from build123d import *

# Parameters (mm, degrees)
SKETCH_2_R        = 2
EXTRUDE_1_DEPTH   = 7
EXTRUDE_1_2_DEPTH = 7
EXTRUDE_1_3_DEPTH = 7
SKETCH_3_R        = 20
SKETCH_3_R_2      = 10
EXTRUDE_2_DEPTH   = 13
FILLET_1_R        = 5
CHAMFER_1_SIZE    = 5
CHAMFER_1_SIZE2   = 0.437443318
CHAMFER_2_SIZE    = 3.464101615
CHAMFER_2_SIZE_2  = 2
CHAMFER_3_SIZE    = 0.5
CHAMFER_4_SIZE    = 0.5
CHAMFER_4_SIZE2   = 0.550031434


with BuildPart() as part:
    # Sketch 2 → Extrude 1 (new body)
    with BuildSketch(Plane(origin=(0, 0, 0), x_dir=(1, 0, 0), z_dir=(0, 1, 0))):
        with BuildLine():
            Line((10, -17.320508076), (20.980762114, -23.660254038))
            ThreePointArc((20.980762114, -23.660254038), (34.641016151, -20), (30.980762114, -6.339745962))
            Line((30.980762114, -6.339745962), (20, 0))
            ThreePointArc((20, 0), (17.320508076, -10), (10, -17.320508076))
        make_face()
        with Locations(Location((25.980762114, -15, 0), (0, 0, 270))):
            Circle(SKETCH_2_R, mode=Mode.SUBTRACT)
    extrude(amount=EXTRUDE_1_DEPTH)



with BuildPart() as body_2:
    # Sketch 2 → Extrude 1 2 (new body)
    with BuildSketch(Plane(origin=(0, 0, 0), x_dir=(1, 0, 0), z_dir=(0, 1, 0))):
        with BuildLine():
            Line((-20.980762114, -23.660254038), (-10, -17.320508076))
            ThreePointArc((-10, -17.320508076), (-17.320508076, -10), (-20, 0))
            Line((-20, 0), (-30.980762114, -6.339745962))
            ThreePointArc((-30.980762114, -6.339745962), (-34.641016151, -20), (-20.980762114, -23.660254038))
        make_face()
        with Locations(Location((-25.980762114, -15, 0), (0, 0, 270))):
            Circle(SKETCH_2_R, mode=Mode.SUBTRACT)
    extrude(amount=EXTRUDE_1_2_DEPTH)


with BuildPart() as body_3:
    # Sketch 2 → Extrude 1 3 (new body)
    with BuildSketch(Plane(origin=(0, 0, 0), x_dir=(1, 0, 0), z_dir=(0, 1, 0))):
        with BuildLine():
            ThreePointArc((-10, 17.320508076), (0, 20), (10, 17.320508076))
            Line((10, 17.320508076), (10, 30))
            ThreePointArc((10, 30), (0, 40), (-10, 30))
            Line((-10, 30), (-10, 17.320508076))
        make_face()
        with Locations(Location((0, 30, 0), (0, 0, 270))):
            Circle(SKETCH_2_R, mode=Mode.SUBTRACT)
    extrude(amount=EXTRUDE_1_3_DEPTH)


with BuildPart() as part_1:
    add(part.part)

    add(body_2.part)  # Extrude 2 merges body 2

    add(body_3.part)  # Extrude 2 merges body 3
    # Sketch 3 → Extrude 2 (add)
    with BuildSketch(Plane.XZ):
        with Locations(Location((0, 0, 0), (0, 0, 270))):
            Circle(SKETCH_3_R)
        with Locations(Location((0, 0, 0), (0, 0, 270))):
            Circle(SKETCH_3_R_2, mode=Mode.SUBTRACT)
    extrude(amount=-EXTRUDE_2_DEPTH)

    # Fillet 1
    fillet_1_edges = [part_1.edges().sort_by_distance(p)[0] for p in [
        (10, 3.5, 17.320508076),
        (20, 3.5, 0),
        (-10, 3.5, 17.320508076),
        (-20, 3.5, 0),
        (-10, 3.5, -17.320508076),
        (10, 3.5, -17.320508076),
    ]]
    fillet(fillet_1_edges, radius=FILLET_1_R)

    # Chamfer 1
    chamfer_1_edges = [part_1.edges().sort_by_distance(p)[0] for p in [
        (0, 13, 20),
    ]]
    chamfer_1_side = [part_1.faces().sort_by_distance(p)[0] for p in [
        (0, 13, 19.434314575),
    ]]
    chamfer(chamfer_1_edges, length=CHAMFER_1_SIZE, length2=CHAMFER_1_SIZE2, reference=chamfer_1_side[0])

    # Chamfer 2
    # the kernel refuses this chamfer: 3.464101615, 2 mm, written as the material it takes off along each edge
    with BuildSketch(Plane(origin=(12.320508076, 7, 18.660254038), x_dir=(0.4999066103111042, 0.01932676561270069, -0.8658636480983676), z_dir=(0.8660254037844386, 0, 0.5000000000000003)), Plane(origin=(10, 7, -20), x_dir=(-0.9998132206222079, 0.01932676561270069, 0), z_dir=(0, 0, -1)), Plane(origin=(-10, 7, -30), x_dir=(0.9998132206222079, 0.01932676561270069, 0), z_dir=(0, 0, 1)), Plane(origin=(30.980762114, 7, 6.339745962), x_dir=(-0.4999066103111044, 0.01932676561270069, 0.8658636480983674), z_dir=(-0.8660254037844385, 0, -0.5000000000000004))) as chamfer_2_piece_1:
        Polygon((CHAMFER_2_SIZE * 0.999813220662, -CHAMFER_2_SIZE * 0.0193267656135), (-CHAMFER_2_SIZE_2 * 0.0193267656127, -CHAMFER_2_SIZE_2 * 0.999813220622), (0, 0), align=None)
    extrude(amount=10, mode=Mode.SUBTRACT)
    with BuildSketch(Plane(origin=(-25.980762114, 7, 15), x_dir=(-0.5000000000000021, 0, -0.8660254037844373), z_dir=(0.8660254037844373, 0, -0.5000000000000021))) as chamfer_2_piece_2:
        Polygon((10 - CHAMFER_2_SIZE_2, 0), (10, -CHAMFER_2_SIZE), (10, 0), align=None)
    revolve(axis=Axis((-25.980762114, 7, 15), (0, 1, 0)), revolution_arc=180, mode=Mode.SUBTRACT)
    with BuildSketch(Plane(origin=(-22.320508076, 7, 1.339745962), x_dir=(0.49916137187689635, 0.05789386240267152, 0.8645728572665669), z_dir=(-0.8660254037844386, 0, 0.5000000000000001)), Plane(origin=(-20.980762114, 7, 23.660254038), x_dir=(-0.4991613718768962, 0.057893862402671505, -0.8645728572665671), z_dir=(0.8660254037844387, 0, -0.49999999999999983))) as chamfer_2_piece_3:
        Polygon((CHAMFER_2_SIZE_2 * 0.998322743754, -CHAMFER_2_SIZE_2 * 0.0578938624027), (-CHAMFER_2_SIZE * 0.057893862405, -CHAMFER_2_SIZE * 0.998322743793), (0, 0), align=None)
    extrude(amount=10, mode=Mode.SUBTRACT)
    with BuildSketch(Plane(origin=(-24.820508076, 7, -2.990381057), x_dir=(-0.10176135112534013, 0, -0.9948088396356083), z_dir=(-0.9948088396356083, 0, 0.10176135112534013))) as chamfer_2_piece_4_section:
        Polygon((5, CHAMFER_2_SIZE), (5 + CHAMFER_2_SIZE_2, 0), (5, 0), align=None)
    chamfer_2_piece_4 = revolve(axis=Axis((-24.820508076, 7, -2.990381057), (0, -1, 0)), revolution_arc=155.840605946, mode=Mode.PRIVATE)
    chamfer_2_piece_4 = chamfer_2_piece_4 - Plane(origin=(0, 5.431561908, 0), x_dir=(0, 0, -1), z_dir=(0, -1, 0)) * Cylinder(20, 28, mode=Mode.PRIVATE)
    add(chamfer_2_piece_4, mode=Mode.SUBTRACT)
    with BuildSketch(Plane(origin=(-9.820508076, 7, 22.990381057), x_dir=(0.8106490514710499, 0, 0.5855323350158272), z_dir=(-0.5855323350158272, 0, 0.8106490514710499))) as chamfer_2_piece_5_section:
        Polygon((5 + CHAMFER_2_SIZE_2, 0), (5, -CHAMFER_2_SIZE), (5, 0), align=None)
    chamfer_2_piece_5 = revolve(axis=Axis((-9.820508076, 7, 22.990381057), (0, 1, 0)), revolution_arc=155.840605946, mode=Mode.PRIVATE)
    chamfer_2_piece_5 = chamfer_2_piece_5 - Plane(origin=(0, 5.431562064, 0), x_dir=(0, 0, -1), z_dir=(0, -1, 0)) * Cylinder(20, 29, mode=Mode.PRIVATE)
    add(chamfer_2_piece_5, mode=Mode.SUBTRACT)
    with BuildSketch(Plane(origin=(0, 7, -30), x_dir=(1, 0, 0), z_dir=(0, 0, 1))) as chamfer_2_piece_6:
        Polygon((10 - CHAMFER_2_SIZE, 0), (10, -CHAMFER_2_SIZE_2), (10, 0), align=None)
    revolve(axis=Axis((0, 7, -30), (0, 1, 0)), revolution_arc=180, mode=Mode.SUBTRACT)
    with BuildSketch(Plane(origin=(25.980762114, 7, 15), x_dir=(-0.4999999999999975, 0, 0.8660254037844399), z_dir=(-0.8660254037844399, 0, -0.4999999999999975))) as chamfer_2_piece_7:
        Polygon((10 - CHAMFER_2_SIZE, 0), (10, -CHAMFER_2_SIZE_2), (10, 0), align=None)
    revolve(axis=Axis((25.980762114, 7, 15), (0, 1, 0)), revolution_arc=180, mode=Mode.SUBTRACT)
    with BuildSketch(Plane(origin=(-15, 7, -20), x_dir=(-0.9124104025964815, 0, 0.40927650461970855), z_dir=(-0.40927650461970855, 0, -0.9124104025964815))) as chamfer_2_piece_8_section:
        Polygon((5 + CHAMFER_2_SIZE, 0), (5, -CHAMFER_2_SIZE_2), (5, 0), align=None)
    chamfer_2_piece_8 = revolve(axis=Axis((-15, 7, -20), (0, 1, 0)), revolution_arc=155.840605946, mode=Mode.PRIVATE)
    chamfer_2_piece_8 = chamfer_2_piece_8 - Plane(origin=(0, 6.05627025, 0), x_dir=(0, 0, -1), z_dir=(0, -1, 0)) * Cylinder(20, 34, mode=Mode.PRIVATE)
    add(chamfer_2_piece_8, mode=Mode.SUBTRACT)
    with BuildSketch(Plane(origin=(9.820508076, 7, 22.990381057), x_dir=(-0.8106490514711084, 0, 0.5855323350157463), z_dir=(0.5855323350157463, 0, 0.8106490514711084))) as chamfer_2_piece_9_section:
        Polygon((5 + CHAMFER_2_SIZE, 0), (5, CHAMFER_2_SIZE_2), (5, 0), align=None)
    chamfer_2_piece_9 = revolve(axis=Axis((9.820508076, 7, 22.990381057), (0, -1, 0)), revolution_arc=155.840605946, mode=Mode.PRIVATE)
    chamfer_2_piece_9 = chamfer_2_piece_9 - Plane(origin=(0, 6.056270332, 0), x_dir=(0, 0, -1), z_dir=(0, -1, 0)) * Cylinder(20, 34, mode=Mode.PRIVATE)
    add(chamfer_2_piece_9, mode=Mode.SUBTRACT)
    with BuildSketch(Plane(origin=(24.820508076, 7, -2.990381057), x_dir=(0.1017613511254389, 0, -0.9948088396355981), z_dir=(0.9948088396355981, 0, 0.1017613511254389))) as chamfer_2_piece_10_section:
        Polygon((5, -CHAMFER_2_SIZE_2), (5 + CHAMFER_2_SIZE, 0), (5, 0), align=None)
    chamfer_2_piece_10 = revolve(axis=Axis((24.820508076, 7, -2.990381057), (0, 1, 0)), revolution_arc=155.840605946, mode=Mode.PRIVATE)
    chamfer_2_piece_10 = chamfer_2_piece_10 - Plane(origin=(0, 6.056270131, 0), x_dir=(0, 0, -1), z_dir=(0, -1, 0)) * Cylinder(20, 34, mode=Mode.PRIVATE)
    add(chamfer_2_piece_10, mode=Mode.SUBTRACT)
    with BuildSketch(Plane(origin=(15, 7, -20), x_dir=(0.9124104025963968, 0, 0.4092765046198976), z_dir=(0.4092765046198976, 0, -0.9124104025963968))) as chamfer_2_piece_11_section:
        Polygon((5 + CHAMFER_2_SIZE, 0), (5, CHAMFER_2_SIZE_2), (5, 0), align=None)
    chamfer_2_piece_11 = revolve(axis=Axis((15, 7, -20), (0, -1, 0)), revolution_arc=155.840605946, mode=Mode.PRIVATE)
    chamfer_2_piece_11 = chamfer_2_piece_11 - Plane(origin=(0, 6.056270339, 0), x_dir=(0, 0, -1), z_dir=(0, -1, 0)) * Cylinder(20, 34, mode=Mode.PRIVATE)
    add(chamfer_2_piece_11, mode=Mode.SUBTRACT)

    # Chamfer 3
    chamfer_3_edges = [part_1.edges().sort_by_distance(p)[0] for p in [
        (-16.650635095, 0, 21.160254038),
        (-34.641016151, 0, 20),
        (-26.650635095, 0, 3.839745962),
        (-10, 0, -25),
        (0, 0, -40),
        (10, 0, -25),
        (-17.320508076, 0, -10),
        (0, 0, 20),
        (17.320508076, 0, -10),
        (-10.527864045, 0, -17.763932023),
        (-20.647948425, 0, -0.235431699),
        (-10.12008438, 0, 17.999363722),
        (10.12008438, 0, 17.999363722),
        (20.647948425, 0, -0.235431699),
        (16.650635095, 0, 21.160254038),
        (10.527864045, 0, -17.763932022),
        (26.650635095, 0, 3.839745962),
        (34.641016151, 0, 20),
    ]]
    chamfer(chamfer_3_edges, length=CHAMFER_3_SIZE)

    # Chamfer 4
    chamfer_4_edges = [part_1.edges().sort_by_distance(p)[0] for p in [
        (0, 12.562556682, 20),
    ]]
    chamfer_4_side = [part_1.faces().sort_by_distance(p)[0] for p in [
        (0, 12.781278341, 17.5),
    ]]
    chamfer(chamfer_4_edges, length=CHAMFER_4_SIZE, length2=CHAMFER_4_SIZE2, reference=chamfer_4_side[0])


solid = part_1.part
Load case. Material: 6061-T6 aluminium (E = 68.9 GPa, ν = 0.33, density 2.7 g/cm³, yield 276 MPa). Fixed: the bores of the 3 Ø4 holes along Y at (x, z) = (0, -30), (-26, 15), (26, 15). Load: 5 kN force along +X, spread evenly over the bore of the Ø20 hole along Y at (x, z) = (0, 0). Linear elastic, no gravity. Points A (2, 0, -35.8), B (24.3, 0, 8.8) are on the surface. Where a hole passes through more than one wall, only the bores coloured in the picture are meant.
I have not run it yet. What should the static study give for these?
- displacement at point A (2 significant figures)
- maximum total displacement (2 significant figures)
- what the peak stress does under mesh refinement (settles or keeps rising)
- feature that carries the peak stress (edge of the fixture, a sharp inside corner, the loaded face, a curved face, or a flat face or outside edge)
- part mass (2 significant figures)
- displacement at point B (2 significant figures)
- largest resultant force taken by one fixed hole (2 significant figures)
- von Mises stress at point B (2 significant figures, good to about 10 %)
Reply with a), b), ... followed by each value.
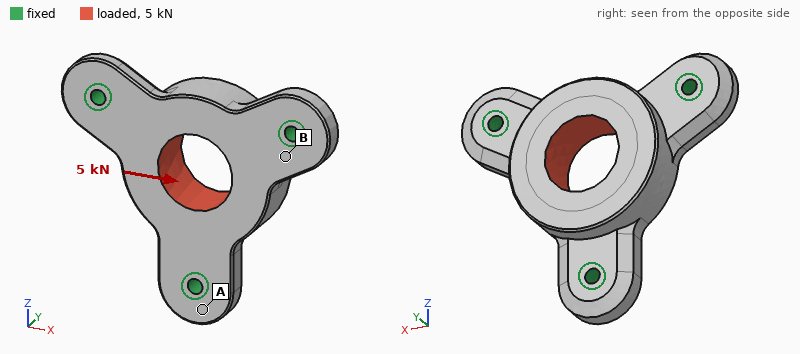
a) 2.8 µm
b) 17 µm
c) keeps rising
d) edge of the fixture
e) 52 g
f) 4.4 µm
g) 2.2 kN
h) 14 MPa
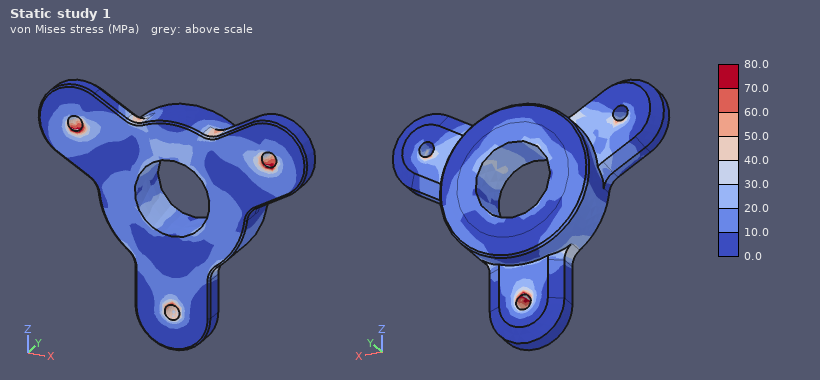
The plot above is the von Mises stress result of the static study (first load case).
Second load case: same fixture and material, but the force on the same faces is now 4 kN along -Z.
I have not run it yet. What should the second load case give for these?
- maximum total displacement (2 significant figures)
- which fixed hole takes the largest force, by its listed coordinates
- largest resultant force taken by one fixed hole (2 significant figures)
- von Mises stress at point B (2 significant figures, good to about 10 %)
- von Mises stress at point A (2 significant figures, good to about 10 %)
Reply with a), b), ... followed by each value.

a) 14 µm
b) (0, -30)
c) 2.0 kN
d) 13 MPa
e) 8.5 MPa
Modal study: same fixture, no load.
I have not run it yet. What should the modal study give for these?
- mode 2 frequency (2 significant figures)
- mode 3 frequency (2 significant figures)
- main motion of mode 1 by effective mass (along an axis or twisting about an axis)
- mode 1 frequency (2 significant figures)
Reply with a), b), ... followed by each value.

a) 15 kHz
b) 15 kHz
c) along Y
d) 12 kHz
